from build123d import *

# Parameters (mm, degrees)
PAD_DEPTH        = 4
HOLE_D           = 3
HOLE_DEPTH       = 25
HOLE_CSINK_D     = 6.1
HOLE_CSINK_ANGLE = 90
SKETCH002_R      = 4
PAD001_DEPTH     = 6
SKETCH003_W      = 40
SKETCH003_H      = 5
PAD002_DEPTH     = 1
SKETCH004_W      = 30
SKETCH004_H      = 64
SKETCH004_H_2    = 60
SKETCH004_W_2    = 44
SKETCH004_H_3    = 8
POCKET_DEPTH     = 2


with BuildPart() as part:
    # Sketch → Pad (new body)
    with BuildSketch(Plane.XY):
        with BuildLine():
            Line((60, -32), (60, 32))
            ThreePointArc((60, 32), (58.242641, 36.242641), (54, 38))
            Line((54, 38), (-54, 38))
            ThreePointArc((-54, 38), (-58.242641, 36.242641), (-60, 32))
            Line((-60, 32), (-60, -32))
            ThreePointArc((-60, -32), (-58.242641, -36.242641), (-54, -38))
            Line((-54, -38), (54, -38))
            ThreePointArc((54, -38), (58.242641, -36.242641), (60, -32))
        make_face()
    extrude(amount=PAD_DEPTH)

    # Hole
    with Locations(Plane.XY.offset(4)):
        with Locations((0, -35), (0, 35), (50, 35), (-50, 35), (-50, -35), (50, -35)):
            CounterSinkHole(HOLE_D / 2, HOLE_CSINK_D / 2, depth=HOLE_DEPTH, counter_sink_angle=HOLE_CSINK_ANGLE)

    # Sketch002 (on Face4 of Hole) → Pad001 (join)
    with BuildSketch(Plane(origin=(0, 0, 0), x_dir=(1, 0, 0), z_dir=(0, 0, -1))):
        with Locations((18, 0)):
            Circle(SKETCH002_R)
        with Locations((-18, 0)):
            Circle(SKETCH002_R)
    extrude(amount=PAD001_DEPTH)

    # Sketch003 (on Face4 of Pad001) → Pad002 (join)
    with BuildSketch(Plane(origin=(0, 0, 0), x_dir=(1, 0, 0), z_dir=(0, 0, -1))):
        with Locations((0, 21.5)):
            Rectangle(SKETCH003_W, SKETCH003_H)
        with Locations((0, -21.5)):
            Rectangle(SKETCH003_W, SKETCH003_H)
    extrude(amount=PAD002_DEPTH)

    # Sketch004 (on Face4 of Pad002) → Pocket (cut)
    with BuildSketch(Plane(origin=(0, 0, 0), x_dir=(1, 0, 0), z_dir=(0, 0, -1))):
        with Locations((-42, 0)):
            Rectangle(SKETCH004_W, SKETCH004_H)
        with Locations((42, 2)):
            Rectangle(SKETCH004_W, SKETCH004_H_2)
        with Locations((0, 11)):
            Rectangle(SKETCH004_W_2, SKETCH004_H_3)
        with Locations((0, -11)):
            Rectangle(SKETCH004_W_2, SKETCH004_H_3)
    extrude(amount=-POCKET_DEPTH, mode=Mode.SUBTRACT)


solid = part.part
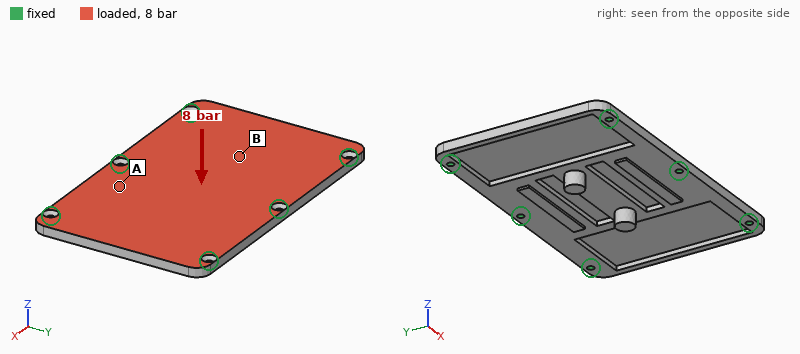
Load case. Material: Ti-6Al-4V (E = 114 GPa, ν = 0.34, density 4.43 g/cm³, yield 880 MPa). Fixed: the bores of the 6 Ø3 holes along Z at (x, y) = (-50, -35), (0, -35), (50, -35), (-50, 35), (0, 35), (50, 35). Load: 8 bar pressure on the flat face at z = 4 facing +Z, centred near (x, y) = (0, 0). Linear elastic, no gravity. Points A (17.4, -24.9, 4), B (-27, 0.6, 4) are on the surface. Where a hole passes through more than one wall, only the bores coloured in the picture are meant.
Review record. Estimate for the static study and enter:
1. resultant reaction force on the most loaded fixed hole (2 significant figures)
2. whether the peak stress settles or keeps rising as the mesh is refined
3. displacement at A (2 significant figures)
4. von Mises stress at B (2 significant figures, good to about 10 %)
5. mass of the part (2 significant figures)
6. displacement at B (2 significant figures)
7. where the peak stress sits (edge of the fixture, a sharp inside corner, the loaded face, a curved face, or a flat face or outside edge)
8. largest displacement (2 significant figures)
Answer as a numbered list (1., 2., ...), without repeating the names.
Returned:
1. 3.6 kN
2. keeps rising
3. 0.14 mm
4. 100 MPa
5. 130 g
6. 0.35 mm
7. edge of the fixture
8. 0.38 mm
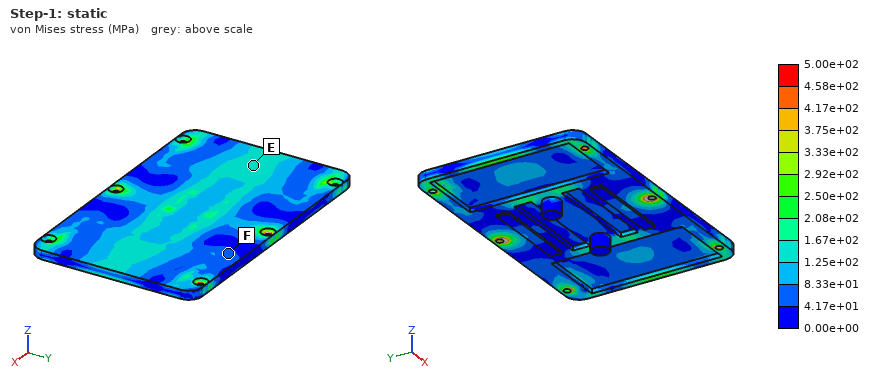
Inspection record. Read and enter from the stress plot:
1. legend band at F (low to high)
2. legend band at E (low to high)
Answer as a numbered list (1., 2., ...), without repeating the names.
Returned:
1. 4.17e+01 to 8.33e+01 MPa
2. 1.25e+02 to 1.67e+02 MPa
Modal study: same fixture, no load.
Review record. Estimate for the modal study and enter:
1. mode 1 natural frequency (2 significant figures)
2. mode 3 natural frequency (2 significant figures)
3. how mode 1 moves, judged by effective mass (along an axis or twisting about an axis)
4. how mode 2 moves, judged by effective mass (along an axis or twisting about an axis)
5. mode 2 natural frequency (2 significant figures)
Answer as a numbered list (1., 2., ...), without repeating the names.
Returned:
1. 2500 Hz
2. 3700 Hz
3. along Z
4. twisting about Y
5. 2900 Hz
